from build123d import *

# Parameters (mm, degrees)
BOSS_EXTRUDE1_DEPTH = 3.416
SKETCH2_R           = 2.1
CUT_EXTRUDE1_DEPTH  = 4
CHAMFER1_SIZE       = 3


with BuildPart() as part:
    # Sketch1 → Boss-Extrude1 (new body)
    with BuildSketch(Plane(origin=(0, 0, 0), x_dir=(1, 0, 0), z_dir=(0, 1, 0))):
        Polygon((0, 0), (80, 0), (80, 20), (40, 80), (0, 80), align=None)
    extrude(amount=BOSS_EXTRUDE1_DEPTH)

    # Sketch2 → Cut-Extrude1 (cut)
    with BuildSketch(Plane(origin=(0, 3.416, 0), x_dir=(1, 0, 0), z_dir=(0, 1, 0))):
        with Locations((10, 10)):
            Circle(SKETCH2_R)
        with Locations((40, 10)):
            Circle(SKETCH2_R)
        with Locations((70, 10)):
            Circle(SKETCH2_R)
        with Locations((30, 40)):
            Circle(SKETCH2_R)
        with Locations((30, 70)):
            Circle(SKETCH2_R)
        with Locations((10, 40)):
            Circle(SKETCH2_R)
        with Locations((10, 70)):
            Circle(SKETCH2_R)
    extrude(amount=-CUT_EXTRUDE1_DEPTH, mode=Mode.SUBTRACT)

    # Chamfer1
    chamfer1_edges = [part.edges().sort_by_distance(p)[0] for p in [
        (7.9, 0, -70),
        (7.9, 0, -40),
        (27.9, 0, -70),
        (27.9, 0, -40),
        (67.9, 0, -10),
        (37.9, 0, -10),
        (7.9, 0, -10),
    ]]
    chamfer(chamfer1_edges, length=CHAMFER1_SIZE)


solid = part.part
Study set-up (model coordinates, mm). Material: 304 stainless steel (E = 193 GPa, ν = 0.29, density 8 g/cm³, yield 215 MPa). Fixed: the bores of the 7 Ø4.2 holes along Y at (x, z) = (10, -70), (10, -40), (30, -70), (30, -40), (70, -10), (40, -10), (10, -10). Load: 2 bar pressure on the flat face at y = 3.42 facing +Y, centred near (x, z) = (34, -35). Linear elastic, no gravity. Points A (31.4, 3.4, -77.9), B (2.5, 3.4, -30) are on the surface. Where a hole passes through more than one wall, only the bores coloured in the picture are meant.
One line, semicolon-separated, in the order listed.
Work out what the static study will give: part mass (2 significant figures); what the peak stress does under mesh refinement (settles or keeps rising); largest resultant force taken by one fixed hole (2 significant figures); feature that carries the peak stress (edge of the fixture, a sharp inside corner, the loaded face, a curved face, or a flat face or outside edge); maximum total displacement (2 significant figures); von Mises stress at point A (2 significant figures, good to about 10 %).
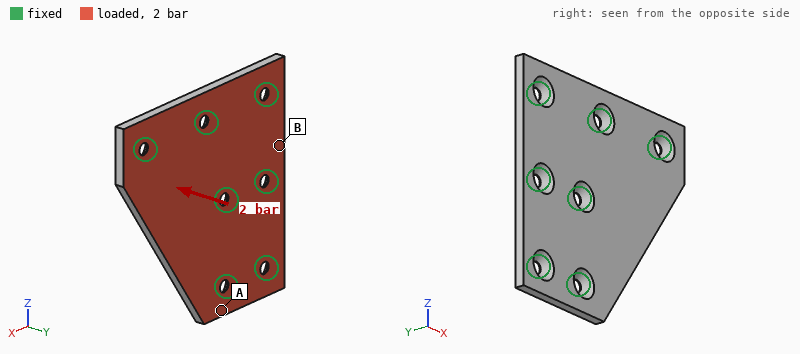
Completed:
130 g; keeps rising; 340 N; edge of the fixture; 27 µm; 16 MPa
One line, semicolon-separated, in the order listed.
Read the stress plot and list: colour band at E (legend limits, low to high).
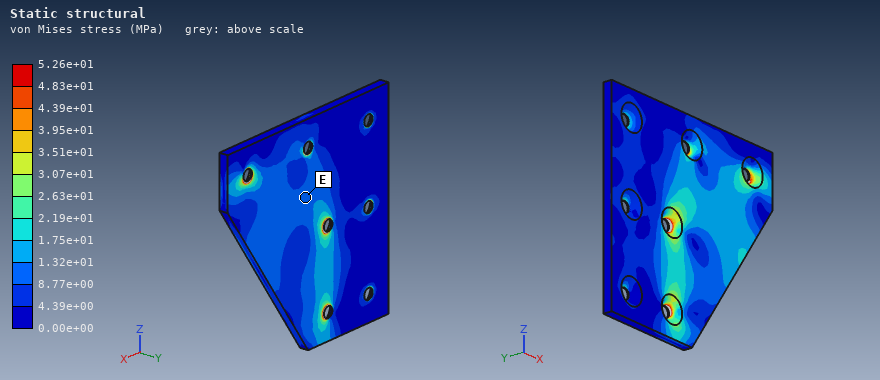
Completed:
8.77e+00 to 1.32e+01 MPa
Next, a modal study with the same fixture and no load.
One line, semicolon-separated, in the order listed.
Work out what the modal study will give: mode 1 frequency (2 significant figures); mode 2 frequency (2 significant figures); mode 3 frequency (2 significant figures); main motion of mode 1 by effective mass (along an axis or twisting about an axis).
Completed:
3400 Hz; 7000 Hz; 10 kHz; along Y
